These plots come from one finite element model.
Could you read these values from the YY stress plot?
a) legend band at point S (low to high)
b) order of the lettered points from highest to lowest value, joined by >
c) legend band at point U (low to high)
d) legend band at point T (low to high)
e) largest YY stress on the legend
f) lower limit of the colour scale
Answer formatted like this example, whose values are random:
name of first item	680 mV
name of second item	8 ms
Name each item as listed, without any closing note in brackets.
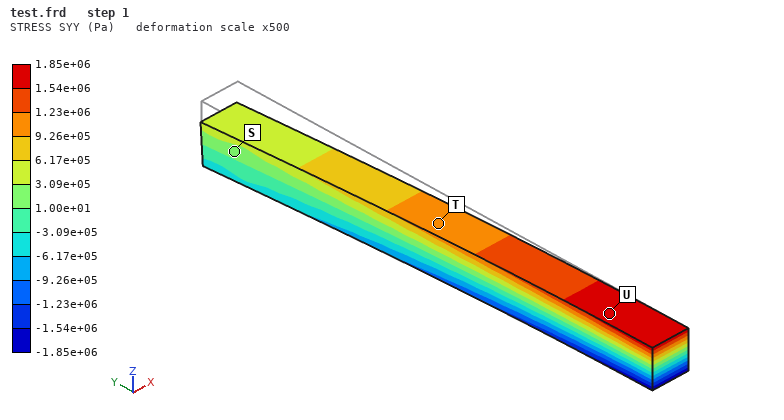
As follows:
legend band at point S	1.00e+01 to 3.09e+05 Pa
order of the lettered points from highest to lowest value, joined by >	U > T > S
legend band at point U	1.54e+06 to 1.85e+06 Pa
legend band at point T	9.26e+05 to 1.23e+06 Pa
largest YY stress on the legend	1.85e+06 Pa
lower limit of the colour scale	-1.85e+06 Pa
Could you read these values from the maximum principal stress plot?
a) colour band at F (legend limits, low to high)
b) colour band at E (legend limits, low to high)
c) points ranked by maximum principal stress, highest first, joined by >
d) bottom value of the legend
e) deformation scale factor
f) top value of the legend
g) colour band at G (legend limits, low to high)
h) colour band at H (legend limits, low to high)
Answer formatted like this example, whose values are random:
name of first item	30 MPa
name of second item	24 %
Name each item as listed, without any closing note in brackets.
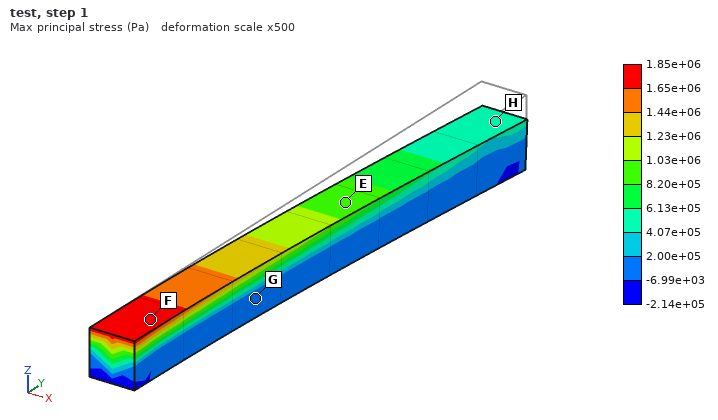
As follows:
colour band at F	1.65e+06 to 1.85e+06 Pa
colour band at E	8.20e+05 to 1.03e+06 Pa
points ranked by maximum principal stress, highest first, joined by >	F > E > H > G
bottom value of the legend	-2.14e+05 Pa
deformation scale factor	500
top value of the legend	1.85e+06 Pa
colour band at G	-6.99e+03 to 2.00e+05 Pa
colour band at H	4.07e+05 to 6.13e+05 Pa
